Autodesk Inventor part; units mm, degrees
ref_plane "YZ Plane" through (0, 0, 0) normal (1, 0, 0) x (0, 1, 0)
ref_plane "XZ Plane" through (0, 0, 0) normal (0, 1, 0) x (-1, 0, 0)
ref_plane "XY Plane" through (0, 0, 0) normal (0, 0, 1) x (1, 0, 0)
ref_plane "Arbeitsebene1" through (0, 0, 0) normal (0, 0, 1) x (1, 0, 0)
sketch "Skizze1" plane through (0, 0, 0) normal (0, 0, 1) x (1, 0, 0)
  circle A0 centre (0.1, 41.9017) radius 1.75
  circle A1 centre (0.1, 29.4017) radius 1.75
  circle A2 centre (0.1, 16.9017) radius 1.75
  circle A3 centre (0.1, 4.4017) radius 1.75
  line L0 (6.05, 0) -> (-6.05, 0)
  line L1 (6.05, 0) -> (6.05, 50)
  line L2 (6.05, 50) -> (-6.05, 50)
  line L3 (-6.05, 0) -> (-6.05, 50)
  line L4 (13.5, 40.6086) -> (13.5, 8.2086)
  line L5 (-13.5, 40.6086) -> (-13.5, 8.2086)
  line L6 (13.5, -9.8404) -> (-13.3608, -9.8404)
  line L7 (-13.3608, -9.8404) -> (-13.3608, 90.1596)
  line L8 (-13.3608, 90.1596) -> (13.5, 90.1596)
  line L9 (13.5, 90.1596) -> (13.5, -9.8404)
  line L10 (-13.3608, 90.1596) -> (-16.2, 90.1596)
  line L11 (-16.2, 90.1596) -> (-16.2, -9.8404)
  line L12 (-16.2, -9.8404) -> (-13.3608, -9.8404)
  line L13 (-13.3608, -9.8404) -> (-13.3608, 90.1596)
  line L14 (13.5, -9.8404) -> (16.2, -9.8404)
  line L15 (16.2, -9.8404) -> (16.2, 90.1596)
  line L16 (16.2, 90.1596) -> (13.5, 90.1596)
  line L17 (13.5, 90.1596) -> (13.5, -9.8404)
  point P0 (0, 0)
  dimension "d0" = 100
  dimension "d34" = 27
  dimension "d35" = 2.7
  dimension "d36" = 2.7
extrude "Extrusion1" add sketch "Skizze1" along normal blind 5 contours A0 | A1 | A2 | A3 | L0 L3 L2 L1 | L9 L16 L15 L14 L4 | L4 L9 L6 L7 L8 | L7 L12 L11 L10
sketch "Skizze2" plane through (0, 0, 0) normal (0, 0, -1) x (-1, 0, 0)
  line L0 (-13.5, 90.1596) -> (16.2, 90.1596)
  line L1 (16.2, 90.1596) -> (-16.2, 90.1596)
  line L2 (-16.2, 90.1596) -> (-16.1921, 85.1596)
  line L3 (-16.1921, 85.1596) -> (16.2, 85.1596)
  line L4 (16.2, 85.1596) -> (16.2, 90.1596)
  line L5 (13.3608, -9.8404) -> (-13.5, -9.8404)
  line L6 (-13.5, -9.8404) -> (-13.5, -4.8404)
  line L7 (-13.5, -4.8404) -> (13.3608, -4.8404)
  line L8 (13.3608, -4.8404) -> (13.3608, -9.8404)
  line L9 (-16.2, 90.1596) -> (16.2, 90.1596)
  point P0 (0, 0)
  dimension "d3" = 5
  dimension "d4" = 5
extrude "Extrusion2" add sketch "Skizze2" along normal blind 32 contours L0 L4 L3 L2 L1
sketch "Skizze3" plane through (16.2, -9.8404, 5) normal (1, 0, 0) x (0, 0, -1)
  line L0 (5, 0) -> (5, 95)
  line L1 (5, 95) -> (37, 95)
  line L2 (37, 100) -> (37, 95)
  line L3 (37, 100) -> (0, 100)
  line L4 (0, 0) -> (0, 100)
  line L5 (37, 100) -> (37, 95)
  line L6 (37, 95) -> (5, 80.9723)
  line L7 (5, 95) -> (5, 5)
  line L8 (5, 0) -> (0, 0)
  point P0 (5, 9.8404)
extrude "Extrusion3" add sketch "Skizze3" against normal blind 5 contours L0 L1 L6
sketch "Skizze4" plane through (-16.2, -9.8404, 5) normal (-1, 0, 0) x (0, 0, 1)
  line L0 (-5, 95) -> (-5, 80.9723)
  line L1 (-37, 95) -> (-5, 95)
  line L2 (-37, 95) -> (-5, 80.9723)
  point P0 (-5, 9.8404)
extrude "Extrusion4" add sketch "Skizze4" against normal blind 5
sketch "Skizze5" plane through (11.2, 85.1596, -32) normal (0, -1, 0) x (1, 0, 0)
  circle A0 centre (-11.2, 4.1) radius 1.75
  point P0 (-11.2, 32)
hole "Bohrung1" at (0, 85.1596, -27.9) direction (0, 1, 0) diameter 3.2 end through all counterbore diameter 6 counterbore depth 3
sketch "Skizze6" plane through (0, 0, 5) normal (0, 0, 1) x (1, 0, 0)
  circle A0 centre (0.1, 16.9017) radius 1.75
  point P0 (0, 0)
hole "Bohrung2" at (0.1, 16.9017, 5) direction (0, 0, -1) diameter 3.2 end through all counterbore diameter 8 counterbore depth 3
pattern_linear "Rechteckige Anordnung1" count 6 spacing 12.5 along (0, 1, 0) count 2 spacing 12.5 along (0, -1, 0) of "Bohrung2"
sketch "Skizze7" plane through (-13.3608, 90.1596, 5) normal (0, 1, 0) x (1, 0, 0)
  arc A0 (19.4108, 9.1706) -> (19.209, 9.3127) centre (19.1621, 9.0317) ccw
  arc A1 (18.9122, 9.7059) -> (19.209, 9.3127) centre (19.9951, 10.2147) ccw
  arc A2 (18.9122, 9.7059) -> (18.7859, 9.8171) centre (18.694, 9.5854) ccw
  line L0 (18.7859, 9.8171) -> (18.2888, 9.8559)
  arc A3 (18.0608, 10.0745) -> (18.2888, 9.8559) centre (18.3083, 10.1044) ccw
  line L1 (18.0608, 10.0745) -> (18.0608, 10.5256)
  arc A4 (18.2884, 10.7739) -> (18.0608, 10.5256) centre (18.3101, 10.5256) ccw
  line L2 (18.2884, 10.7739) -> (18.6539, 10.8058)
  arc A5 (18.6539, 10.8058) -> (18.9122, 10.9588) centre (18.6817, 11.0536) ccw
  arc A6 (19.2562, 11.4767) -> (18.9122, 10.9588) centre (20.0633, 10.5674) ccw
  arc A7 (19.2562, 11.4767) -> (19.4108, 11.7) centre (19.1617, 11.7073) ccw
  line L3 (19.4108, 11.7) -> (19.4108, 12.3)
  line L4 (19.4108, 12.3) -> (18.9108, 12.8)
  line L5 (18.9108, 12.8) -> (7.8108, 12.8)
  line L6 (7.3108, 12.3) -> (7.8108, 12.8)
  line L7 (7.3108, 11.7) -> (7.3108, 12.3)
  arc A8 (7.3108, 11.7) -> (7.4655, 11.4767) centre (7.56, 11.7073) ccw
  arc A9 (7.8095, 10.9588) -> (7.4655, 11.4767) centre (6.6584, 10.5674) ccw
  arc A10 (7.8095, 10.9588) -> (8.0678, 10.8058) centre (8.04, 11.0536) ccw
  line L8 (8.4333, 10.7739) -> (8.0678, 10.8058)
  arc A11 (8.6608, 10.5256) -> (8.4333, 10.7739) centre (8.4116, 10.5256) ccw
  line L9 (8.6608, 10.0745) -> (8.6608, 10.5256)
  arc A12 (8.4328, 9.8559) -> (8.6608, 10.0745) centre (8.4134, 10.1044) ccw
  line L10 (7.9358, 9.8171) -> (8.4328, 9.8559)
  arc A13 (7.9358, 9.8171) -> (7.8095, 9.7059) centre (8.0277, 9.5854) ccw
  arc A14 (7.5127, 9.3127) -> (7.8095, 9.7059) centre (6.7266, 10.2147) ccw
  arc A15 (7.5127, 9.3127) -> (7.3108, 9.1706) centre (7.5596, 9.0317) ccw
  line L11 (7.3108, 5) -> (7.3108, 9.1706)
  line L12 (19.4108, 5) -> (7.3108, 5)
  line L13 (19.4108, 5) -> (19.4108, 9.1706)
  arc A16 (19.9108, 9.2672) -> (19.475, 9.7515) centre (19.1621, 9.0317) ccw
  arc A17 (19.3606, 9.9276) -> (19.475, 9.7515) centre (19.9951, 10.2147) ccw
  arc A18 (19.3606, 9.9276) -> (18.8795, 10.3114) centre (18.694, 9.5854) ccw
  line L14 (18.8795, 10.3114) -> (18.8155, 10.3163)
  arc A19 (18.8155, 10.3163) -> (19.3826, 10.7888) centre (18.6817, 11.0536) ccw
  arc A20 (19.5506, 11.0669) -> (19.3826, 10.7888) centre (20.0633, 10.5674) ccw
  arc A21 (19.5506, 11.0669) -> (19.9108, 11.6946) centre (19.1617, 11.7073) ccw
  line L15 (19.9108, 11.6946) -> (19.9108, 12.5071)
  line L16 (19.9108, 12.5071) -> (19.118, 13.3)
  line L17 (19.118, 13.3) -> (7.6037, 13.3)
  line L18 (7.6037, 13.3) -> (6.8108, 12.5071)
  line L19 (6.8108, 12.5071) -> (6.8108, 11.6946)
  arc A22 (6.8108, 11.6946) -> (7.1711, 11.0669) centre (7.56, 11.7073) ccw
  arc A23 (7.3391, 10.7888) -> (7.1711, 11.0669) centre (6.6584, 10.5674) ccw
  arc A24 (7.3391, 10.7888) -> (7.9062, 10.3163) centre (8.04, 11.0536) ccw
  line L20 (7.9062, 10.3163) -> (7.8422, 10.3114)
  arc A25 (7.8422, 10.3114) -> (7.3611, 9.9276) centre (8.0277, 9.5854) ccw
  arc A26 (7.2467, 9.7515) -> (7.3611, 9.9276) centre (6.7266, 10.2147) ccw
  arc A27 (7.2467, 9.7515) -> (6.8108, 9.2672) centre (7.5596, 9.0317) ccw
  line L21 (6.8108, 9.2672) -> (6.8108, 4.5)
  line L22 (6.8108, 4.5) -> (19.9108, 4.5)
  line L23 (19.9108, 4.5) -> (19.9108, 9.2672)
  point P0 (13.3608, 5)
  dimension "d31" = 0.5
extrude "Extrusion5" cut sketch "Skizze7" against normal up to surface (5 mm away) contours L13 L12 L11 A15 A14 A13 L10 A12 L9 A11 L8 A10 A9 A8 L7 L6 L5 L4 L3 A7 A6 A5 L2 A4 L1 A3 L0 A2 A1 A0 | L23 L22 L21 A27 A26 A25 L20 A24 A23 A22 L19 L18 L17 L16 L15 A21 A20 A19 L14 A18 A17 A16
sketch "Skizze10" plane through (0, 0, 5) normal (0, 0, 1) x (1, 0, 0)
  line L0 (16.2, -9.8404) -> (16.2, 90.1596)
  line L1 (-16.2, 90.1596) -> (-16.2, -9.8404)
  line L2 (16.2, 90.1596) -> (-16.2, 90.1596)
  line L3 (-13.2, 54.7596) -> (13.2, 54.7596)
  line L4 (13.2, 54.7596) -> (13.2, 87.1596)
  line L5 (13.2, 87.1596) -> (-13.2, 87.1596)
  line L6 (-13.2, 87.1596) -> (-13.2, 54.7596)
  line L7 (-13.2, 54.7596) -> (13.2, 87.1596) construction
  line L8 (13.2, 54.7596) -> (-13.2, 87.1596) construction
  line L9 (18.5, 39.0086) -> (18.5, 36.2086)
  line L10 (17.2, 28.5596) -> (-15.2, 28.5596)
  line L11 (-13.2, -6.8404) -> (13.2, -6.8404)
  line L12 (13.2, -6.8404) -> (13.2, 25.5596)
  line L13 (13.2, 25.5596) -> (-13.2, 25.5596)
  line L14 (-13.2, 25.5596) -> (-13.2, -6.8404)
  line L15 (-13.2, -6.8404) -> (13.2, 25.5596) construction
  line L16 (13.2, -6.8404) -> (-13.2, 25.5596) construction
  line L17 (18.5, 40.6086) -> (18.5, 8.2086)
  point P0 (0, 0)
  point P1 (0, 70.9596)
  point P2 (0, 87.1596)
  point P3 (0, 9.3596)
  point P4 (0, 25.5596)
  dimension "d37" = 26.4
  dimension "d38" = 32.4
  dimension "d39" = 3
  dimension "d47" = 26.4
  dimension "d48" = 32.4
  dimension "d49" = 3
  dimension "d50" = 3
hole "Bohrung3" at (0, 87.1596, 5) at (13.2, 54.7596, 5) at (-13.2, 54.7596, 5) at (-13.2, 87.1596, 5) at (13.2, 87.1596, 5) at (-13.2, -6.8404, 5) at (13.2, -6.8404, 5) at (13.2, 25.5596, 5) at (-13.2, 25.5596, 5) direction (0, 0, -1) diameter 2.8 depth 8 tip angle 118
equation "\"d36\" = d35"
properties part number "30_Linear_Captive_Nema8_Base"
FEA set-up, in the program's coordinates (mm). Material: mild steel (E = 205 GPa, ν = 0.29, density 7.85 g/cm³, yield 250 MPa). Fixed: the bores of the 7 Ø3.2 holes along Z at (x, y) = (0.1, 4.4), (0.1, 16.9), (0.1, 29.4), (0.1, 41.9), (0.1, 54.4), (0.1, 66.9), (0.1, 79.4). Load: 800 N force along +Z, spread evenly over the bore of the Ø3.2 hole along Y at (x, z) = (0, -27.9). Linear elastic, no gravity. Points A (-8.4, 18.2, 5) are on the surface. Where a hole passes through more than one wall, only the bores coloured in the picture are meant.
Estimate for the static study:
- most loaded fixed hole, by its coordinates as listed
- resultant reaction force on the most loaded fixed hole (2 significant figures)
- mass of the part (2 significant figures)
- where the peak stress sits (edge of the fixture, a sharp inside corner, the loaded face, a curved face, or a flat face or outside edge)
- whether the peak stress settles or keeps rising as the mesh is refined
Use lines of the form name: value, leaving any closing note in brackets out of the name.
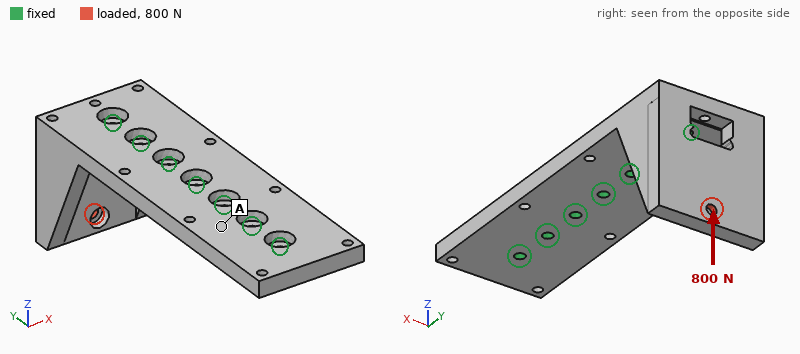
most loaded fixed hole, by its coordinates as listed: (0.1, 79.4)
resultant reaction force on the most loaded fixed hole: 1.2 kN
mass of the part: 170 g
where the peak stress sits: edge of the fixture
whether the peak stress settles or keeps rising as the mesh is refined: keeps rising
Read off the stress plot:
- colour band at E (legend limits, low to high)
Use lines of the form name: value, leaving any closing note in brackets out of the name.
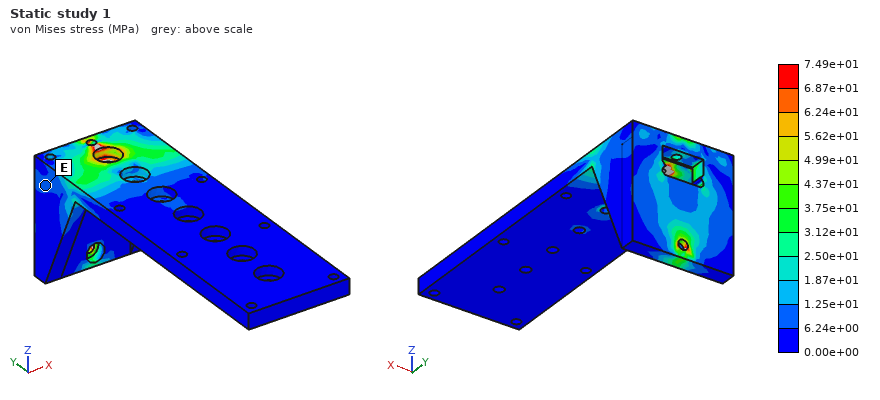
colour band at E: 6.24e+00 to 1.25e+01 MPa
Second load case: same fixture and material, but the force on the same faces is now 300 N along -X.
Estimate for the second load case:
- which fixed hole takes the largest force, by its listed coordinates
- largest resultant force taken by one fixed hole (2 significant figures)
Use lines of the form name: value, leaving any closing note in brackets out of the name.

which fixed hole takes the largest force, by its listed coordinates: (0.1, 79.4)
largest resultant force taken by one fixed hole: 350 N
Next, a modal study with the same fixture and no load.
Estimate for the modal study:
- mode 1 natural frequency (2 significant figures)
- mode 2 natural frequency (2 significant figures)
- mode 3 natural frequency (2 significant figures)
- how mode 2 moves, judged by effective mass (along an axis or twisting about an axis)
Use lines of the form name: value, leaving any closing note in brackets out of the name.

mode 1 natural frequency: 2200 Hz
mode 2 natural frequency: 3500 Hz
mode 3 natural frequency: 6000 Hz
how mode 2 moves, judged by effective mass: along Y
